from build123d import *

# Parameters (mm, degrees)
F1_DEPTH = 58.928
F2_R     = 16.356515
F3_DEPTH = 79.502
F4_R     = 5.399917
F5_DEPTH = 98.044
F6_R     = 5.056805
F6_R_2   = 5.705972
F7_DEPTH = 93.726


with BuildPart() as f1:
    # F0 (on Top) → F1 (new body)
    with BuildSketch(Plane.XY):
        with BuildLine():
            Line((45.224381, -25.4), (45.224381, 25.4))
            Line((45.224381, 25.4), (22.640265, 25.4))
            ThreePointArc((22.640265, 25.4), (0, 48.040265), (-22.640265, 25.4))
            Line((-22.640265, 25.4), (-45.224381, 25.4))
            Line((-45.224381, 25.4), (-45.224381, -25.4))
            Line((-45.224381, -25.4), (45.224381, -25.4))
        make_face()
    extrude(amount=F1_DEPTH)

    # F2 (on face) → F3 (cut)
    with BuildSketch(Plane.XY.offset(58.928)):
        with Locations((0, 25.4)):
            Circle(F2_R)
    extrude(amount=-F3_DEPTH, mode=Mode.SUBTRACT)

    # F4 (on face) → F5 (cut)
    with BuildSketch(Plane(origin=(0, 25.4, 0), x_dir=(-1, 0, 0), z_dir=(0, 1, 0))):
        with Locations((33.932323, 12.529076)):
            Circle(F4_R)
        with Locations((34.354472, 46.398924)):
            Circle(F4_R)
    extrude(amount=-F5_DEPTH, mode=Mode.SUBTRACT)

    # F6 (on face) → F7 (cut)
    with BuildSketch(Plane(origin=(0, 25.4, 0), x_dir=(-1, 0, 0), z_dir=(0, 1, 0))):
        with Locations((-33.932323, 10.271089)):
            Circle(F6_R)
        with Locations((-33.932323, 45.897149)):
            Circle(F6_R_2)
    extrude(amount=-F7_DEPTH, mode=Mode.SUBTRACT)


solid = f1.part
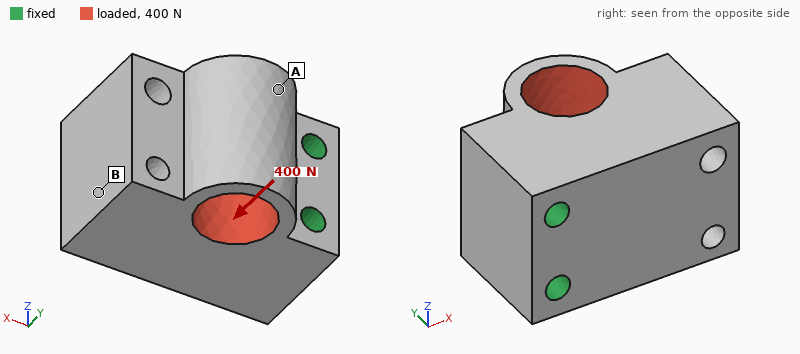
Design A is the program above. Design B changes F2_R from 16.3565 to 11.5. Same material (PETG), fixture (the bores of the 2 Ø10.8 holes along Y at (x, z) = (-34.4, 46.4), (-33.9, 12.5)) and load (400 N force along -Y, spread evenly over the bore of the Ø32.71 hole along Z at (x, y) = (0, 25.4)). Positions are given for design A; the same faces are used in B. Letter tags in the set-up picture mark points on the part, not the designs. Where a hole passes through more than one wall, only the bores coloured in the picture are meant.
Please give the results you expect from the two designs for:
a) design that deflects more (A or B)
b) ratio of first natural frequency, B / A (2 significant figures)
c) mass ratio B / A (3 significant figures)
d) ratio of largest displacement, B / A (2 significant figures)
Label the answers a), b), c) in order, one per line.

a) A
b) 1.1
c) 1.10
d) 0.68
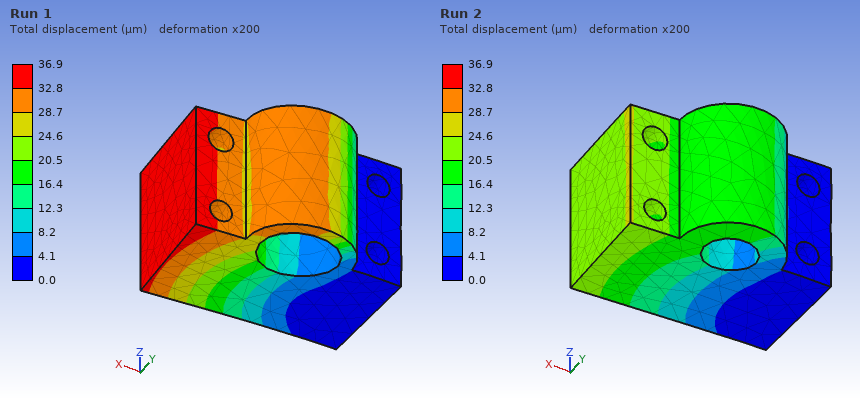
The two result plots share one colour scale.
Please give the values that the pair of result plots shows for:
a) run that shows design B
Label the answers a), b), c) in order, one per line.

a) Run 2
